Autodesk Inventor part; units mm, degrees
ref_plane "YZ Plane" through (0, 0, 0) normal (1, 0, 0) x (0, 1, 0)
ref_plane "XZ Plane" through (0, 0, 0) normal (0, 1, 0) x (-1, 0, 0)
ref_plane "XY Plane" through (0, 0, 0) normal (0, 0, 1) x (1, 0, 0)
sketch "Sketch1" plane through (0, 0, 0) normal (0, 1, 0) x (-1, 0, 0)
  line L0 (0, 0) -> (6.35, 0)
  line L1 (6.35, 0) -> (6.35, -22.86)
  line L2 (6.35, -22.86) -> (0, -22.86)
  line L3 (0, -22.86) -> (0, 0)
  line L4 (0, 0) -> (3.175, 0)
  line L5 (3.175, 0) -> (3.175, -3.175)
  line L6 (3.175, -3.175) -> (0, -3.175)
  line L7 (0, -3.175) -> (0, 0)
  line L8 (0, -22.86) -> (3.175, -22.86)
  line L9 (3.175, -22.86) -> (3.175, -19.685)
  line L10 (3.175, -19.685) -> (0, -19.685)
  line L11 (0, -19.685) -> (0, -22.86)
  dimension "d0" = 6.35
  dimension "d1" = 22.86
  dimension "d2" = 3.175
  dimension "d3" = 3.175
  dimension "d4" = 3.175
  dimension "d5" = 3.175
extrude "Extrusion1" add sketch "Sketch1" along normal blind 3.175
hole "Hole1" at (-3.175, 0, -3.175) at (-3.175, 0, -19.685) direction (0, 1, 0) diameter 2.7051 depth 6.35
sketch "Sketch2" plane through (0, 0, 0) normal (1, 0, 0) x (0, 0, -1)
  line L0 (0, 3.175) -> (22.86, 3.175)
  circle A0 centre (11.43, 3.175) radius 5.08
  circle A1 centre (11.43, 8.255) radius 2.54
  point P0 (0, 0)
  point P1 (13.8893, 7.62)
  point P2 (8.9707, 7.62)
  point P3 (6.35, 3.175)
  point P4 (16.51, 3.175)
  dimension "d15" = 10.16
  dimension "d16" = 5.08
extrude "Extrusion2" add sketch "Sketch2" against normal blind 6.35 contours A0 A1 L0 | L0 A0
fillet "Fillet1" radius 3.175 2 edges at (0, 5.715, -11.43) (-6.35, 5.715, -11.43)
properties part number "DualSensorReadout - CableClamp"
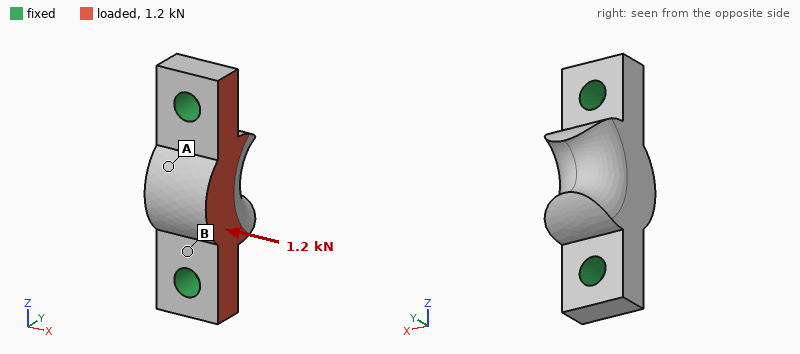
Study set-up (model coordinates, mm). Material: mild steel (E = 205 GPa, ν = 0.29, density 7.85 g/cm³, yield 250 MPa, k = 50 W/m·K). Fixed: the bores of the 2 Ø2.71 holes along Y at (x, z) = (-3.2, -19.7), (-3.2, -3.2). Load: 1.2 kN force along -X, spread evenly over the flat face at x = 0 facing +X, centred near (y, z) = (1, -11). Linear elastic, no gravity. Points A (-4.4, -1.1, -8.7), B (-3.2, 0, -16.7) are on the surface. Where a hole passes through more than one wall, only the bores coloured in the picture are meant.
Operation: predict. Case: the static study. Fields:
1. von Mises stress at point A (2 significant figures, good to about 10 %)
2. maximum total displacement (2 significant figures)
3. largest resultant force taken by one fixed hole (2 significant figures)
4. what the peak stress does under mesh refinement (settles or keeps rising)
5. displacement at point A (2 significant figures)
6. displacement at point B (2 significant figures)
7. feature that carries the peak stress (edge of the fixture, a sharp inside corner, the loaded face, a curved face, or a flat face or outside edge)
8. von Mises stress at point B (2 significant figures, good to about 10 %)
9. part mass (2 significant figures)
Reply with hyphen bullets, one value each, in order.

- 19 MPa
- 2.7 µm
- 600 N
- keeps rising
- 2.1 µm
- 0.93 µm
- edge of the fixture
- 49 MPa
- 5.2 g
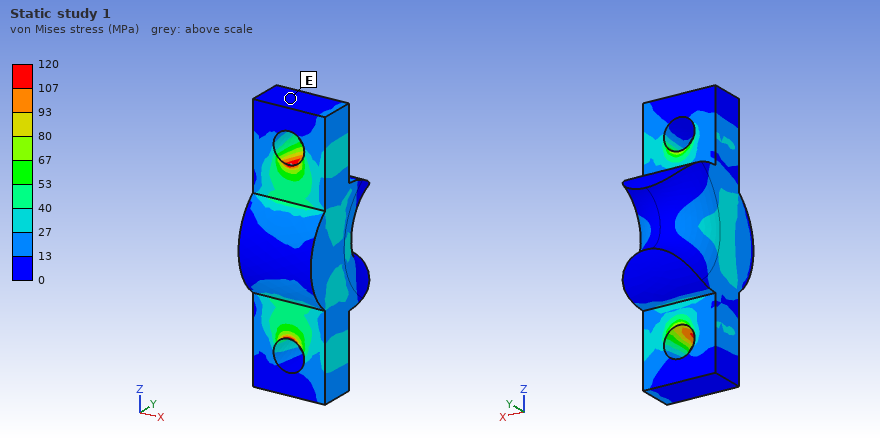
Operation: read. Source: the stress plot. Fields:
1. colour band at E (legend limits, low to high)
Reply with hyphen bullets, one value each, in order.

- 0 to 13 MPa
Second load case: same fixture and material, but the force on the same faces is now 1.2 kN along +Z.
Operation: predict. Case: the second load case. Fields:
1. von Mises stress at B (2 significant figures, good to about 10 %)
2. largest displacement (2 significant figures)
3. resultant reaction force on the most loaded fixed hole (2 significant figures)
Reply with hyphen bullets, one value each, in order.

- 29 MPa
- 1.1 µm
- 630 N
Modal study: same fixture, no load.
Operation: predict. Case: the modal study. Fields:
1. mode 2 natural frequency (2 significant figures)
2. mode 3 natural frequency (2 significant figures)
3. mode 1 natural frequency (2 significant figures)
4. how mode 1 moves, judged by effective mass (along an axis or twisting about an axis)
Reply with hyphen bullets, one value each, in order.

- 56 kHz
- 58 kHz
- 45 kHz
- along X
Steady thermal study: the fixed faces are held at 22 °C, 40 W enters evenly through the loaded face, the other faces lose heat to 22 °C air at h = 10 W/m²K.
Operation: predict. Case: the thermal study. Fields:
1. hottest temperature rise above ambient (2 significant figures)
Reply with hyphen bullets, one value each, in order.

- 74 K
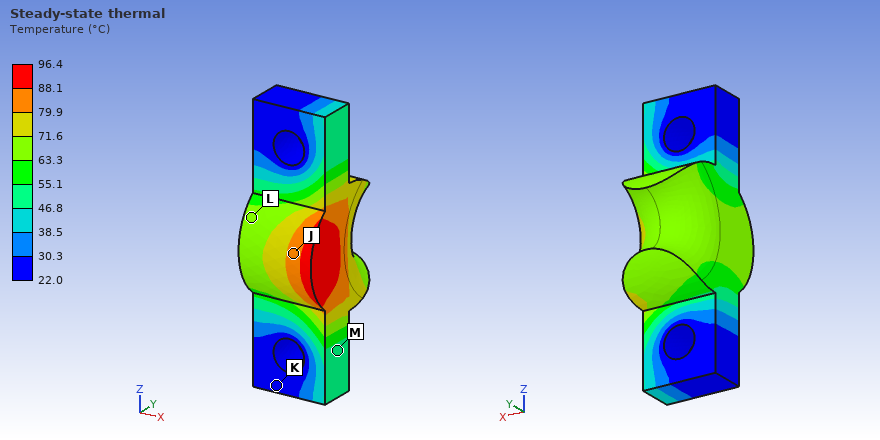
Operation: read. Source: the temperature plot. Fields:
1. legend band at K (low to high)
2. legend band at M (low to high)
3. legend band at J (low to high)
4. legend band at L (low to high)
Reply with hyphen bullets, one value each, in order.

- 22.0 to 30.3 °C
- 46.8 to 55.1 °C
- 79.9 to 88.1 °C
- 63.3 to 71.6 °C
